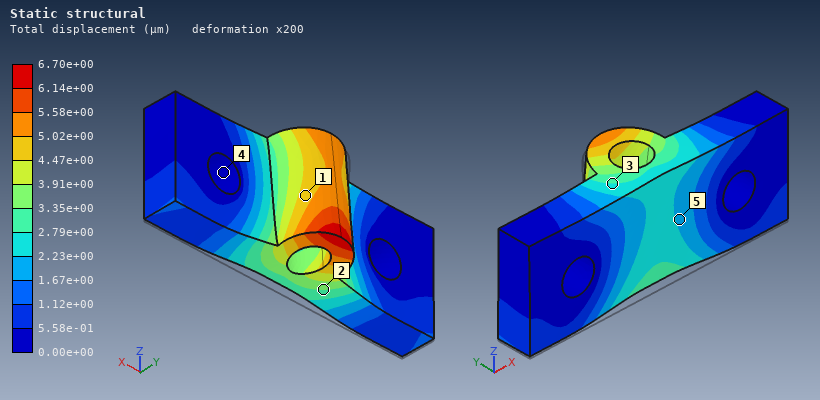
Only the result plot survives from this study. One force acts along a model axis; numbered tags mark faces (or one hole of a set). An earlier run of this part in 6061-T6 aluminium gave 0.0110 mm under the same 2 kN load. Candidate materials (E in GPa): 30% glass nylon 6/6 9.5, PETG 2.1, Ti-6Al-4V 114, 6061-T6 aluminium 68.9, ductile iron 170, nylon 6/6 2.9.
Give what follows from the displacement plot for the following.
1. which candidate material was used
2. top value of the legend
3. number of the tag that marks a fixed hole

Ti-6Al-4V
6.70e+00 µm
4
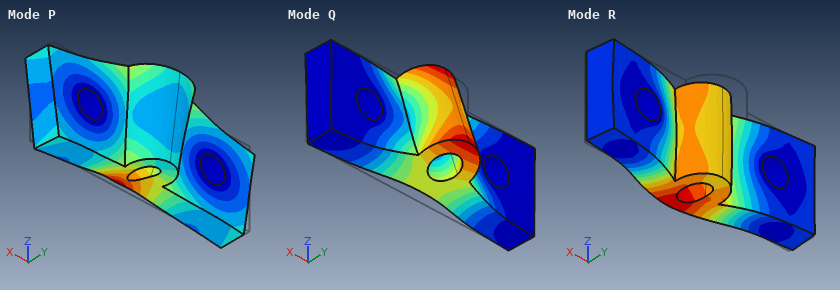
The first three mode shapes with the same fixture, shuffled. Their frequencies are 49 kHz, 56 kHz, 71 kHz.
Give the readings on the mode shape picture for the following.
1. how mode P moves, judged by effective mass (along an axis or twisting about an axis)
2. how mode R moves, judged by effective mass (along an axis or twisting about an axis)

along Z
along Y
